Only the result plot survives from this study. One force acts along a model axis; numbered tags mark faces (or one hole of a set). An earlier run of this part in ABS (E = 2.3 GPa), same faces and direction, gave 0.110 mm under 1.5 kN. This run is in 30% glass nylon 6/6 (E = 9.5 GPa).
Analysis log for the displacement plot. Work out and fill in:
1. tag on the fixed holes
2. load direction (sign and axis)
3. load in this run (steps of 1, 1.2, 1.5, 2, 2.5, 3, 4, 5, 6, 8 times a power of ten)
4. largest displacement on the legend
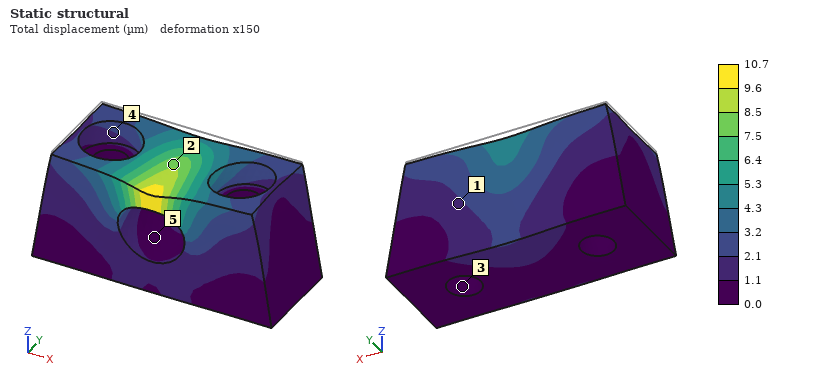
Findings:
3
-Z
600 N
10.7 µm
